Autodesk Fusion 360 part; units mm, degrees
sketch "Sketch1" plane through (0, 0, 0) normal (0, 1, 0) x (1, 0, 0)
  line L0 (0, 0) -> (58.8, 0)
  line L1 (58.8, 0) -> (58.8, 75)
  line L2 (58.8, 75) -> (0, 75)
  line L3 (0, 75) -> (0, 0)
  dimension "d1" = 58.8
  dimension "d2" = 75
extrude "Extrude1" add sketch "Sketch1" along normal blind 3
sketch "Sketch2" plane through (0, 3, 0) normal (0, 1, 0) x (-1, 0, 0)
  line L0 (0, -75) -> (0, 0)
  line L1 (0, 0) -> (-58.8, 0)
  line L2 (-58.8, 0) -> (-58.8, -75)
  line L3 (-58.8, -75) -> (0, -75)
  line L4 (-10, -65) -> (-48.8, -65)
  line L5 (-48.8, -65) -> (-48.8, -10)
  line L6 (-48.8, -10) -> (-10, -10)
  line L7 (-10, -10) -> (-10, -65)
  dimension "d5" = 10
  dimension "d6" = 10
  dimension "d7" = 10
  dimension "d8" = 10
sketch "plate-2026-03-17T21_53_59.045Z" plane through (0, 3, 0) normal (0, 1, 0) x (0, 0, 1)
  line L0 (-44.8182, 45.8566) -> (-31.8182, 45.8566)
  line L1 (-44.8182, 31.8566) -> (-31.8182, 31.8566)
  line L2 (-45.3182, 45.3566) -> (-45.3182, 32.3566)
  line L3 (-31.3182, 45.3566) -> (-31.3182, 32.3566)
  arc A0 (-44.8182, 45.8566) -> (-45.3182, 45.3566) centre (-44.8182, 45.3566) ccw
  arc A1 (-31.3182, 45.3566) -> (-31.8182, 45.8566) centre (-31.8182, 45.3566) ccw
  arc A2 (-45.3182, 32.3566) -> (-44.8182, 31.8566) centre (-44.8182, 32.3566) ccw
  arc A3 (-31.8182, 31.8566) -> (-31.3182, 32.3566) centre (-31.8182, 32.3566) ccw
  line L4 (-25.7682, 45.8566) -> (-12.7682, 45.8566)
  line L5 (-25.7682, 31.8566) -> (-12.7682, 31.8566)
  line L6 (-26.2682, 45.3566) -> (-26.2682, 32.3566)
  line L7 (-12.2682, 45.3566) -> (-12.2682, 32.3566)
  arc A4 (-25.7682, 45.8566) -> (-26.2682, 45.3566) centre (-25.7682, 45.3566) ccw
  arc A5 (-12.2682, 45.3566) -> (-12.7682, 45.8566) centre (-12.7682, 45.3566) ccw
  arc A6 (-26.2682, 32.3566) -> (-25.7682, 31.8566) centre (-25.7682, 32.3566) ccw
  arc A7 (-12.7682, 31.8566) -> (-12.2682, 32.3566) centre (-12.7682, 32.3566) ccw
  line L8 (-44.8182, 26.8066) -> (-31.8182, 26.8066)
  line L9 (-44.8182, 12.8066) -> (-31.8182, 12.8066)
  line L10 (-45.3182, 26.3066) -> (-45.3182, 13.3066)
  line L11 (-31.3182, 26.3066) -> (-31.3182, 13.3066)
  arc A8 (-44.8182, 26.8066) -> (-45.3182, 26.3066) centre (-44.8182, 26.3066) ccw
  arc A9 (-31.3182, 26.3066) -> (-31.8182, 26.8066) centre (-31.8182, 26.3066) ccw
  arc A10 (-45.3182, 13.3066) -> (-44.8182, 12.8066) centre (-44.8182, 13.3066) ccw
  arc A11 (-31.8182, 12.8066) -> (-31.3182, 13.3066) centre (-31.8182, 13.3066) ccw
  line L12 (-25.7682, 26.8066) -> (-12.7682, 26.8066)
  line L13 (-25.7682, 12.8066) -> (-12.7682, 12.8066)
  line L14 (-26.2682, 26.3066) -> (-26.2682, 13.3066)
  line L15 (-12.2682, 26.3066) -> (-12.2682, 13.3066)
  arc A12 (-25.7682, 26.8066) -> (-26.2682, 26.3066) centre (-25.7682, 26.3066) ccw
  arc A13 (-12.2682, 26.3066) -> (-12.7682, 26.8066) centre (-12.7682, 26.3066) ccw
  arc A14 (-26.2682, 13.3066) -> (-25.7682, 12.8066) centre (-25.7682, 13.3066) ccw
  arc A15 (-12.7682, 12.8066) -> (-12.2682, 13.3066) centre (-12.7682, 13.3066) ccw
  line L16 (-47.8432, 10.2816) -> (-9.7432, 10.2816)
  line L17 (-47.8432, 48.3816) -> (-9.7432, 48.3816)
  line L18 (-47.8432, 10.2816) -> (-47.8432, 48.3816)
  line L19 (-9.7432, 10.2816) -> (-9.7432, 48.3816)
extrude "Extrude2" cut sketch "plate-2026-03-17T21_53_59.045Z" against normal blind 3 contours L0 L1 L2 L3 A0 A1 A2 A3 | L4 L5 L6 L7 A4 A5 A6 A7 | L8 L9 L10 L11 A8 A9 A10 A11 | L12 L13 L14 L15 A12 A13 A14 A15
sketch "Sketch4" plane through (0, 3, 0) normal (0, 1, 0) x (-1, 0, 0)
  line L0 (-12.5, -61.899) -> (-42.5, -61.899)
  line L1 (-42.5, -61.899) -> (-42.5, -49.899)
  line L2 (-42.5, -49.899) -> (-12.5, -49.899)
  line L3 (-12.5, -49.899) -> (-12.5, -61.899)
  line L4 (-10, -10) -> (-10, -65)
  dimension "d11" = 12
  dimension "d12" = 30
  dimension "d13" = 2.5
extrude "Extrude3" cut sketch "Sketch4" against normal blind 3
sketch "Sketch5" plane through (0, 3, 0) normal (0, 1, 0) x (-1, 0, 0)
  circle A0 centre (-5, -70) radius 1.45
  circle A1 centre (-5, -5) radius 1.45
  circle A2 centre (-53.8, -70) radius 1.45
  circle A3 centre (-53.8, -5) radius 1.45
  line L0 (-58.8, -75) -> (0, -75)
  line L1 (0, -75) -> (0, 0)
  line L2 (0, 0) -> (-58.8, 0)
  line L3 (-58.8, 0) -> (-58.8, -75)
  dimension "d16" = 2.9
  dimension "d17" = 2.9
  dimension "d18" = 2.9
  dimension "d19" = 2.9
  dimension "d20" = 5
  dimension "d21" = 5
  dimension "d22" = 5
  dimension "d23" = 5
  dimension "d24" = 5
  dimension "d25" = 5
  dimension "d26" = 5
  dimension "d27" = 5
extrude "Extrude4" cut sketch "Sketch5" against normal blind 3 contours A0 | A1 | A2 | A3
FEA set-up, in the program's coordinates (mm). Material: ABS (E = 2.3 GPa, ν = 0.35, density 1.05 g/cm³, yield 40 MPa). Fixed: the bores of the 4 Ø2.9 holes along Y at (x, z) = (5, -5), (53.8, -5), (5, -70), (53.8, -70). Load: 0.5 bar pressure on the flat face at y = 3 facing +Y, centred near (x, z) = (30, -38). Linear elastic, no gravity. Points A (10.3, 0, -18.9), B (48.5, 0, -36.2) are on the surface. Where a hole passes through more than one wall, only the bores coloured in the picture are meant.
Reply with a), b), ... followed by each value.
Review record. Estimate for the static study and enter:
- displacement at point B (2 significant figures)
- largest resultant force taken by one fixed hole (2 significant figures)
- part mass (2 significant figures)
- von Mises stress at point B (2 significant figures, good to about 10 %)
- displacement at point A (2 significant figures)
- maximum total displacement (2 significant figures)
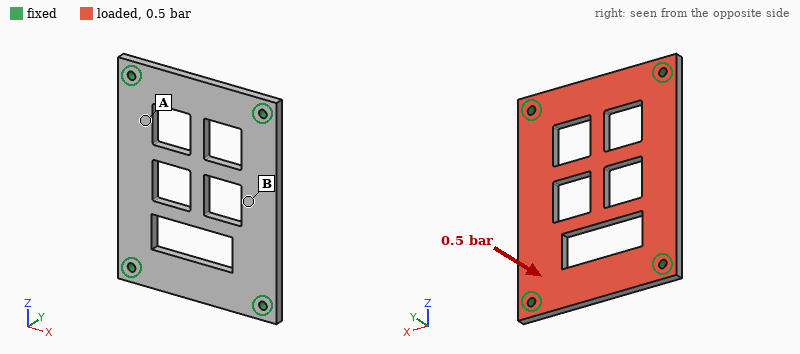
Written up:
a) 0.62 mm
b) 42 N
c) 10 g
d) 7.3 MPa
e) 0.32 mm
f) 0.81 mm
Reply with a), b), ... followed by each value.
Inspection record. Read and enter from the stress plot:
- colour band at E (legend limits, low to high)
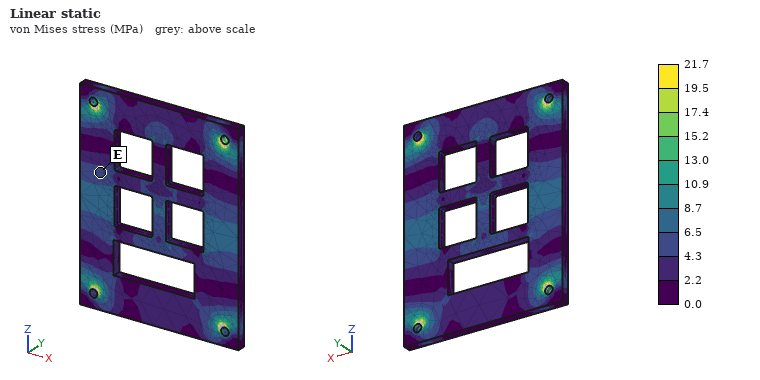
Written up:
a) 4.3 to 6.5 MPa
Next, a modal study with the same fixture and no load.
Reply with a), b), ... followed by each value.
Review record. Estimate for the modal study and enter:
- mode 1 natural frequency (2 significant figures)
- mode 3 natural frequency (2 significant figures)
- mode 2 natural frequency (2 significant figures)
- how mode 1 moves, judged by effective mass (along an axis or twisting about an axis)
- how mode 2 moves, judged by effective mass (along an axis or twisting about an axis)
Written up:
a) 880 Hz
b) 1700 Hz
c) 1200 Hz
d) along Y
e) twisting about Z
